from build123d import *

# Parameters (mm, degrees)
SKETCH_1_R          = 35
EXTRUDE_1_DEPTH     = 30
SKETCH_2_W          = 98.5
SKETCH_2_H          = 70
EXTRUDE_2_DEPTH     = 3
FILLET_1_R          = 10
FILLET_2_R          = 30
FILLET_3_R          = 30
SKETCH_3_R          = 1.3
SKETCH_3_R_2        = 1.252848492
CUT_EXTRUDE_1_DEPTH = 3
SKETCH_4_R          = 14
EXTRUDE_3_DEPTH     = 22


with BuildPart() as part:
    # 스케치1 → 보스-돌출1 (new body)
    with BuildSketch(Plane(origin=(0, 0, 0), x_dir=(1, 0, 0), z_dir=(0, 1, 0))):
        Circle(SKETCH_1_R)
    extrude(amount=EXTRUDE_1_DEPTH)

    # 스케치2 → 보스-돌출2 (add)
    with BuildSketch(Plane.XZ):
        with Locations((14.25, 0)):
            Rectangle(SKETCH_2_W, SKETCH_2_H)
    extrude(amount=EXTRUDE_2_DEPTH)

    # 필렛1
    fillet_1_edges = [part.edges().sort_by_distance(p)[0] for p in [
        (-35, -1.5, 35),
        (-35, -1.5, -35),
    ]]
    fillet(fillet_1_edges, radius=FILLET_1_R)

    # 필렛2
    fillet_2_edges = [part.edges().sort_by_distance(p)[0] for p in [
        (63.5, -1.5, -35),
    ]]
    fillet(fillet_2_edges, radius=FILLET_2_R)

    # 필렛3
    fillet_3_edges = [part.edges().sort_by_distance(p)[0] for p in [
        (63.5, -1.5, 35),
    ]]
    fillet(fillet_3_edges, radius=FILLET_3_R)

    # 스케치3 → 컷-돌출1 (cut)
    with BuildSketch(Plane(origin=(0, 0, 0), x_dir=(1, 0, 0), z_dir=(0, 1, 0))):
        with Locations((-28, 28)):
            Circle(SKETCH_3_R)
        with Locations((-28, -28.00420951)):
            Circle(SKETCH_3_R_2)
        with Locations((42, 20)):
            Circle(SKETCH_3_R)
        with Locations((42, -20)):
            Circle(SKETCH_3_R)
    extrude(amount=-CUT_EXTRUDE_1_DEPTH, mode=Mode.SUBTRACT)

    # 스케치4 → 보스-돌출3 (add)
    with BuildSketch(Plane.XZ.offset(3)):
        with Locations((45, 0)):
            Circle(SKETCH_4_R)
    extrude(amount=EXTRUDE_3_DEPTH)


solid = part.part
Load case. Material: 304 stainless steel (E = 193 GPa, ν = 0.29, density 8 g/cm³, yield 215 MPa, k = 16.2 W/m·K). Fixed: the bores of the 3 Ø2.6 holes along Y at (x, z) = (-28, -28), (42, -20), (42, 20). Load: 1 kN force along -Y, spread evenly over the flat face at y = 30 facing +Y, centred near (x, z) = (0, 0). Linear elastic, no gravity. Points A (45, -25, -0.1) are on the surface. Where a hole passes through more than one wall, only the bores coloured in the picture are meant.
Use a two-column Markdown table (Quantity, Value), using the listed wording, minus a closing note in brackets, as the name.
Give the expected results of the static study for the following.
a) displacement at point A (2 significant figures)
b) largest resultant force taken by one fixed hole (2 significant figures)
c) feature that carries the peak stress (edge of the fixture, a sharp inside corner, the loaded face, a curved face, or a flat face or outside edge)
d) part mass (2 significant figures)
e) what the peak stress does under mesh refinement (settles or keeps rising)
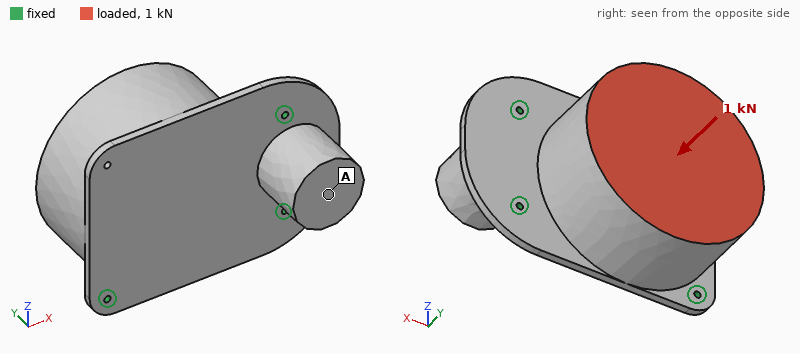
| Quantity | Value |
|---|---|
| displacement at point A | 8.3 µm |
| largest resultant force taken by one fixed hole | 630 N |
| feature that carries the peak stress | edge of the fixture |
| part mass | 1.2 kg |
| what the peak stress does under mesh refinement | keeps rising |
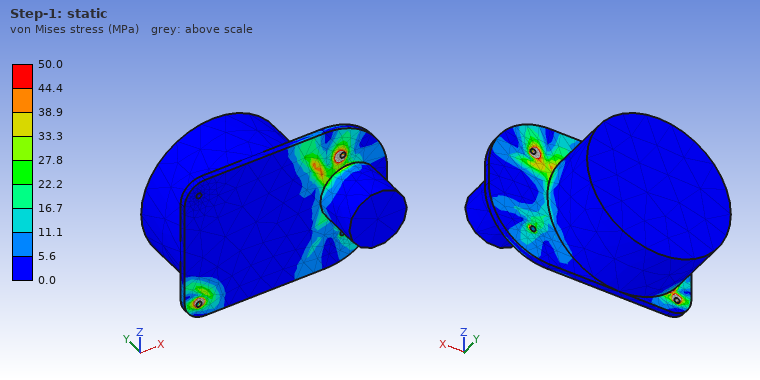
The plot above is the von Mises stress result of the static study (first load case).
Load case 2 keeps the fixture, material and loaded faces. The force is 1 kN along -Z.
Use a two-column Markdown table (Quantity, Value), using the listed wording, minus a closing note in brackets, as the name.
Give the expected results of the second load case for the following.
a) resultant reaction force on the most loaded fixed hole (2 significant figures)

| Quantity | Value |
|---|---|
| resultant reaction force on the most loaded fixed hole | 900 N |
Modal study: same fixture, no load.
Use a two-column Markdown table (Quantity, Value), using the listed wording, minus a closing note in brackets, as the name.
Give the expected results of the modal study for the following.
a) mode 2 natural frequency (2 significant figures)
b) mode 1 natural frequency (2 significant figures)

| Quantity | Value |
|---|---|
| mode 2 natural frequency | 2500 Hz |
| mode 1 natural frequency | 1000 Hz |
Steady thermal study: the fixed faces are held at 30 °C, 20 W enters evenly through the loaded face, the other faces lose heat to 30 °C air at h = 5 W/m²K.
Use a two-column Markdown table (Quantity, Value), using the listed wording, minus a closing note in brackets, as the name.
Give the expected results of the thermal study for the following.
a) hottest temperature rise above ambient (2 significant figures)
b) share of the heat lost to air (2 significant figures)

| Quantity | Value |
|---|---|
| hottest temperature rise above ambient | 76 K |
| share of the heat lost to air | 25 % |
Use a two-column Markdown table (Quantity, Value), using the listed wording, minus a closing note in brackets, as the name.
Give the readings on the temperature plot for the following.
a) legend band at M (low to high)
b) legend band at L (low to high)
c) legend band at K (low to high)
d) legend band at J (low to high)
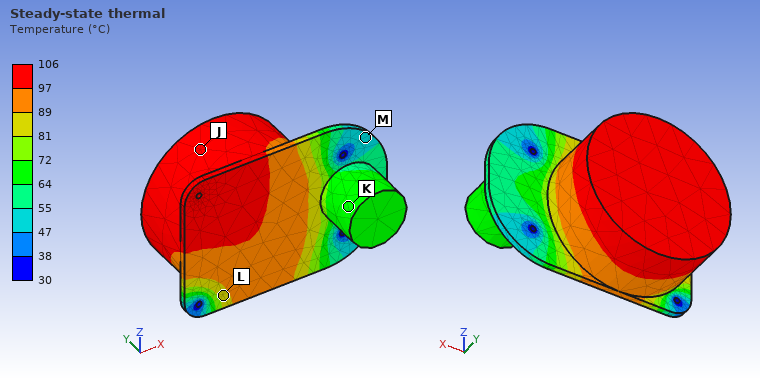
| Quantity | Value |
|---|---|
| legend band at M | 47 to 55 °C |
| legend band at L | 81 to 89 °C |
| legend band at K | 64 to 72 °C |
| legend band at J | 97 to 106 °C |
